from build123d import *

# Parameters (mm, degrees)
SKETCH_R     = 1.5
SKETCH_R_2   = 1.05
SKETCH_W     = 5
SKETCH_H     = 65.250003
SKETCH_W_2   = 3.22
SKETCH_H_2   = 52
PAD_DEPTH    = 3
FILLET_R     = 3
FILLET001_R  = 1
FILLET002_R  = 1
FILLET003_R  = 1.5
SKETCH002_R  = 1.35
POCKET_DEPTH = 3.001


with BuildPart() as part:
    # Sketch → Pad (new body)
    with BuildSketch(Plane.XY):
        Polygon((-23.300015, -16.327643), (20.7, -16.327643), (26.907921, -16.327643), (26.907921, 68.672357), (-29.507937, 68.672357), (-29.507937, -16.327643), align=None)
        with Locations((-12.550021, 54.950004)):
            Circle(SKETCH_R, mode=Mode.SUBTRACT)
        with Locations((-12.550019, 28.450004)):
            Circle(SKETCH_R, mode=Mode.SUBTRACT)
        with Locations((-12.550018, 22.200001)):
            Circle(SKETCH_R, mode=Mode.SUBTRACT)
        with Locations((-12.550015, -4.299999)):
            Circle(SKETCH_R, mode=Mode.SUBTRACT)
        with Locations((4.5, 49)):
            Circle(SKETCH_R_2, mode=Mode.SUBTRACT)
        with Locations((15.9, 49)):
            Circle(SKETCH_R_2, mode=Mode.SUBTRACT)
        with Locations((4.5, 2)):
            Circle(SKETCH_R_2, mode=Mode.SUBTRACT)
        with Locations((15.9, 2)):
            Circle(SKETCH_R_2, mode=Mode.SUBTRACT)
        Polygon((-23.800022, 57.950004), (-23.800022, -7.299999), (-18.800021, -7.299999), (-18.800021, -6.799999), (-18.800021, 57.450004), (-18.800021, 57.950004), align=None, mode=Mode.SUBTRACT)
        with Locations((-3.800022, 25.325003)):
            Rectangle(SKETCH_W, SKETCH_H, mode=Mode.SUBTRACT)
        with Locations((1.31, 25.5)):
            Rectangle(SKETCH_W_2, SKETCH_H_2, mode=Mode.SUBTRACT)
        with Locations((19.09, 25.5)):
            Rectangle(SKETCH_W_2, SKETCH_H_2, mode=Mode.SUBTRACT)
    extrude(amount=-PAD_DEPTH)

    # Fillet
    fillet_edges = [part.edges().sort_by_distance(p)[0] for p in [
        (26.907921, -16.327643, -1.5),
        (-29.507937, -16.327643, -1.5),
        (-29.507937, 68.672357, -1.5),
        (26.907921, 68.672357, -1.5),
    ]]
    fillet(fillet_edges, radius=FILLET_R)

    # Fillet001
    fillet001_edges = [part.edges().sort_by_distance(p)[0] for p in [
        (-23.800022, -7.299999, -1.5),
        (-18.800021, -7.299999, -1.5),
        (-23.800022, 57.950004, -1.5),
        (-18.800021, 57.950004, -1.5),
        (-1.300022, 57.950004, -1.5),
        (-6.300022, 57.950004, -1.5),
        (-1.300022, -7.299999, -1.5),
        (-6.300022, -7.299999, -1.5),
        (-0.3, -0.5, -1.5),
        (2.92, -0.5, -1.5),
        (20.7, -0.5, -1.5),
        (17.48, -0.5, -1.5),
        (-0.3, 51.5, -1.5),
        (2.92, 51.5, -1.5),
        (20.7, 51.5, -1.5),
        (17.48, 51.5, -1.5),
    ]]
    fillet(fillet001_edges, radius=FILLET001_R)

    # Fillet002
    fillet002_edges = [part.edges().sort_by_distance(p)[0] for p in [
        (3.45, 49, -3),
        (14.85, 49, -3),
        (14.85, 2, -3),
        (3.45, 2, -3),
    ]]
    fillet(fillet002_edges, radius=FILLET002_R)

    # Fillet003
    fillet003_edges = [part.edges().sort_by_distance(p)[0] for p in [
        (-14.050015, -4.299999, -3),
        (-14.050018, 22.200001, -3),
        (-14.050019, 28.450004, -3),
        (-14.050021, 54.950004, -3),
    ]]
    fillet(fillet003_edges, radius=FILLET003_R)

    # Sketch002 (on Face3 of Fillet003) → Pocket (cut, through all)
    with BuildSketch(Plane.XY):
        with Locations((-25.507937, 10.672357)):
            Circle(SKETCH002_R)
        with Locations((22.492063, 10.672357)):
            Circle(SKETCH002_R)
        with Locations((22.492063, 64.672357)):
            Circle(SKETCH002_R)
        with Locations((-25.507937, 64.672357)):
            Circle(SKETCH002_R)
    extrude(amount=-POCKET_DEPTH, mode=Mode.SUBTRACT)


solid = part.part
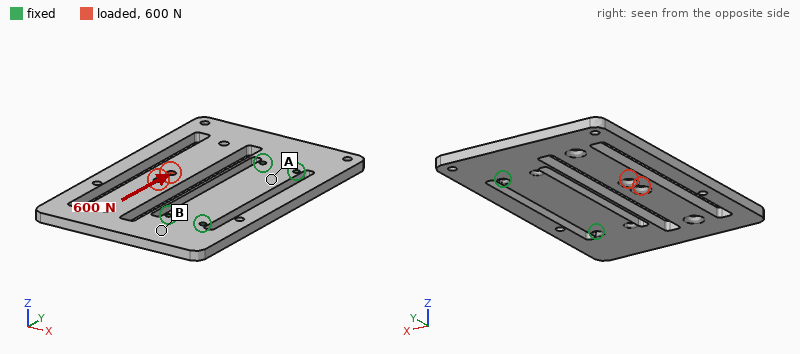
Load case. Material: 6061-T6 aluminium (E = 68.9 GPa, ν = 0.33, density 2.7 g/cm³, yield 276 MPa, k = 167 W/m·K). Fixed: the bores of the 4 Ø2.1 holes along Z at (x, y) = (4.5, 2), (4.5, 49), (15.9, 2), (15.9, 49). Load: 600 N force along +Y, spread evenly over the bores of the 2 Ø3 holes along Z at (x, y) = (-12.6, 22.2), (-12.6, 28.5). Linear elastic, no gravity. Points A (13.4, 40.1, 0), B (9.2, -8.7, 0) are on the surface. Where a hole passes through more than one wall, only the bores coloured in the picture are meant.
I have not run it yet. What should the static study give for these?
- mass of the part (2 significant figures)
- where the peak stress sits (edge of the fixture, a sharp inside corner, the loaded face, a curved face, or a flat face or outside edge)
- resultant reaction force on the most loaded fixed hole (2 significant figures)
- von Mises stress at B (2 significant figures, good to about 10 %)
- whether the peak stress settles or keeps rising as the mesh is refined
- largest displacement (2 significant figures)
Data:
30 g
edge of the fixture
590 N
11 MPa
keeps rising
42 µm
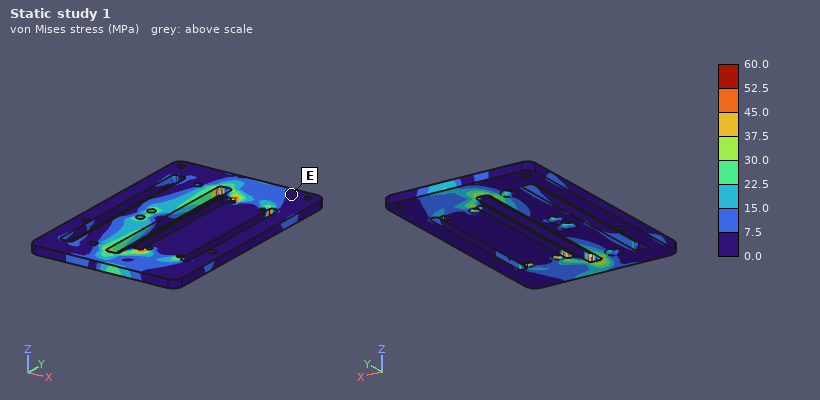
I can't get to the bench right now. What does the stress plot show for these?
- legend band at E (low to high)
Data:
0.0 to 7.5 MPa
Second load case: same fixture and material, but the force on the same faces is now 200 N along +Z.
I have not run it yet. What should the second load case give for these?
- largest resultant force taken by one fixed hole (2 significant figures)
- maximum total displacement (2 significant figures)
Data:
240 N
0.64 mm
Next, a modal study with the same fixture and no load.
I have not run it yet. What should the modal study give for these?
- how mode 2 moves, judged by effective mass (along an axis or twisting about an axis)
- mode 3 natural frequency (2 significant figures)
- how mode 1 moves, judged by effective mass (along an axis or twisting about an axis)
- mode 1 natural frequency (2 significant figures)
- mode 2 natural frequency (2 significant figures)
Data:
twisting about X
1900 Hz
along Z
900 Hz
1700 Hz
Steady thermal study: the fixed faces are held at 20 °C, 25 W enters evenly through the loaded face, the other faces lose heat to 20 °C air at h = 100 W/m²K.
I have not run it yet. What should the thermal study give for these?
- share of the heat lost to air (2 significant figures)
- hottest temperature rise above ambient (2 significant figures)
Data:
63 %
78 K
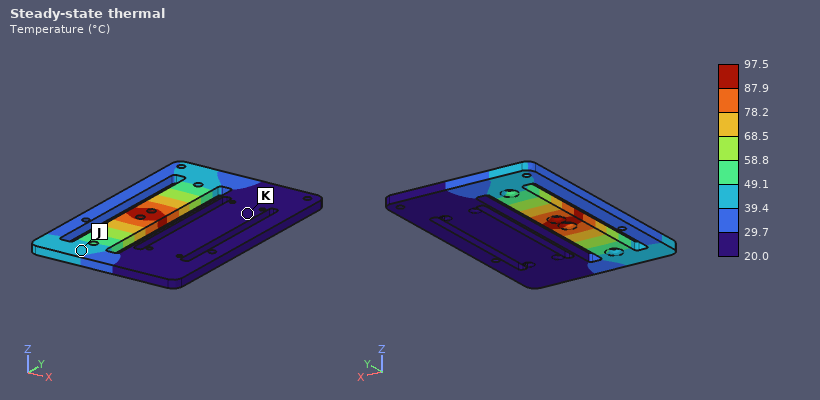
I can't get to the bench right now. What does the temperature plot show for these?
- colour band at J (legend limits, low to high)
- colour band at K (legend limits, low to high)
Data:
39.4 to 49.1 °C
20.0 to 29.7 °C
